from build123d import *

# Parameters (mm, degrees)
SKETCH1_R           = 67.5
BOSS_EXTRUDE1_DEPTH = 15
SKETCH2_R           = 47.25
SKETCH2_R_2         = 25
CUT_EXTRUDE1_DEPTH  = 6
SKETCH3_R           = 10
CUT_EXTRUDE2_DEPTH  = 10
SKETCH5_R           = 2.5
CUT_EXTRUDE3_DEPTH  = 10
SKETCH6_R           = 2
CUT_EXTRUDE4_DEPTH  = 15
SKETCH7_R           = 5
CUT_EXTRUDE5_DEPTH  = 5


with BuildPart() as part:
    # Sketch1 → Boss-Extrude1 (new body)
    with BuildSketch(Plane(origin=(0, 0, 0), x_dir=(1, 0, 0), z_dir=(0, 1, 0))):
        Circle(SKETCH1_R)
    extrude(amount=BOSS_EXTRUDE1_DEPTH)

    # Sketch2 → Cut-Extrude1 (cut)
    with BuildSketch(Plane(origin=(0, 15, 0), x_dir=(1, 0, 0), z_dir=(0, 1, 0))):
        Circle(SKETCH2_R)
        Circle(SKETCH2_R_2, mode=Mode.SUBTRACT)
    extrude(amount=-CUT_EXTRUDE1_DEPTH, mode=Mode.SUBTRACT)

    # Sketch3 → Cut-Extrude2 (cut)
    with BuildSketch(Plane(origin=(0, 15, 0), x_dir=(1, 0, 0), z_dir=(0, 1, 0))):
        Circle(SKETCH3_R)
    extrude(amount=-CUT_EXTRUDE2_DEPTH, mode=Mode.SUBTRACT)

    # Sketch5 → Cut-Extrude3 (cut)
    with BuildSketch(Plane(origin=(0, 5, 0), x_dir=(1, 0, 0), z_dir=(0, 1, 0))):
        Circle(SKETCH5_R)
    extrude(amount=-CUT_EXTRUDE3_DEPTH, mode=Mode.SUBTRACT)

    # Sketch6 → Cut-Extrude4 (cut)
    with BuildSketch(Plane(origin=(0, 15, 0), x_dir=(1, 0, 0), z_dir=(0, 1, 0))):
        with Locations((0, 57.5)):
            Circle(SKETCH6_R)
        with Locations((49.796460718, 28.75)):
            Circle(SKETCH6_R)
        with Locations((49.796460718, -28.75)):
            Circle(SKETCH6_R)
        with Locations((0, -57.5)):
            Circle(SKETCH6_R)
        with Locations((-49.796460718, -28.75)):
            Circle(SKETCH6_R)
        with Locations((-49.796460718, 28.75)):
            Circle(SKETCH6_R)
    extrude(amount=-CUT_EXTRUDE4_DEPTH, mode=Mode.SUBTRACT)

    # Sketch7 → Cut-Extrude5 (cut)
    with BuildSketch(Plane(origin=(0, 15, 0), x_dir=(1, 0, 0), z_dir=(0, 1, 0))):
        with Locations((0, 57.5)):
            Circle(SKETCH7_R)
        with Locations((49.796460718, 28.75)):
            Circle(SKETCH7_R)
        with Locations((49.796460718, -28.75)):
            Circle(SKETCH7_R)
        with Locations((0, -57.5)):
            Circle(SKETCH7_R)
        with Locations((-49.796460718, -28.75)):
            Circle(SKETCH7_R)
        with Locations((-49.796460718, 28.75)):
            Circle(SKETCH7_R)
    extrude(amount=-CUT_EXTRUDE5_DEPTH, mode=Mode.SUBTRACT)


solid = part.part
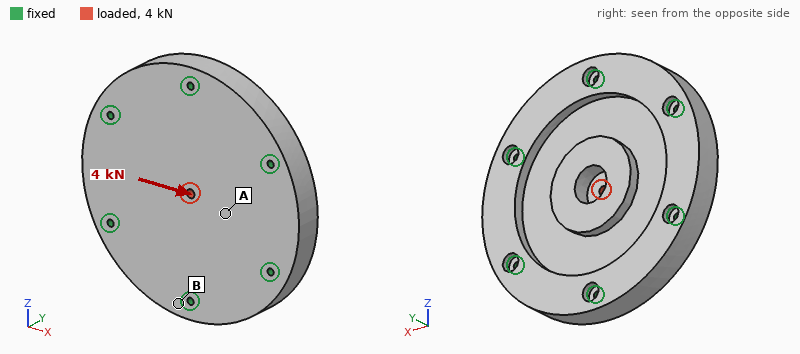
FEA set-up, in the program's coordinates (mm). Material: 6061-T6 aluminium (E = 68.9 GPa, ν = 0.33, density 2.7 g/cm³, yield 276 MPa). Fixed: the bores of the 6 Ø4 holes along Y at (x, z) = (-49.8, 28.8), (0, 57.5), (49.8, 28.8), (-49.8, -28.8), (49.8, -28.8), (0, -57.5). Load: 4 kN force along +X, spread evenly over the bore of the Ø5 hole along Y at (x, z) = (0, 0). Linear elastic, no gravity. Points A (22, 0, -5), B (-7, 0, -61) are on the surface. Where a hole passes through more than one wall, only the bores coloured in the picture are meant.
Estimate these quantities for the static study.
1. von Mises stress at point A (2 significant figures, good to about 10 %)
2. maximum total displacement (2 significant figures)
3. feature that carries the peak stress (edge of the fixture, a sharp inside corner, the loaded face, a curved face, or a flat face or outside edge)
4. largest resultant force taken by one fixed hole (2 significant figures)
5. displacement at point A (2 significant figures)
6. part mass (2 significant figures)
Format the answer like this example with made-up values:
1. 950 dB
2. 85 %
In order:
1. 7.5 MPa
2. 8.4 µm
3. the loaded face
4. 850 N
5. 2.6 µm
6. 480 g
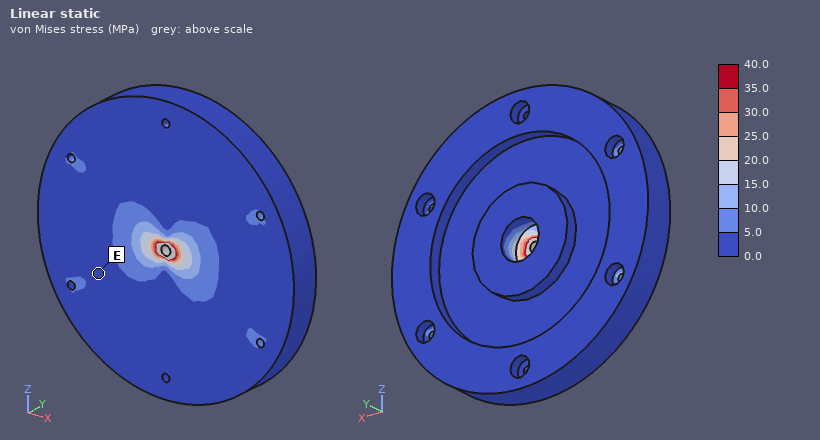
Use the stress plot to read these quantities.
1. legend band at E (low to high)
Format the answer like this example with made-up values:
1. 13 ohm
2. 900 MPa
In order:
1. 0.0 to 5.0 MPa
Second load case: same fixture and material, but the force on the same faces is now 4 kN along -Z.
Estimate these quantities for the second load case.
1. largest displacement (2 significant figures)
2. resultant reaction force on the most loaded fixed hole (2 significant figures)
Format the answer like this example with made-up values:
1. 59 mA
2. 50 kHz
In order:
1. 8.4 µm
2. 960 N
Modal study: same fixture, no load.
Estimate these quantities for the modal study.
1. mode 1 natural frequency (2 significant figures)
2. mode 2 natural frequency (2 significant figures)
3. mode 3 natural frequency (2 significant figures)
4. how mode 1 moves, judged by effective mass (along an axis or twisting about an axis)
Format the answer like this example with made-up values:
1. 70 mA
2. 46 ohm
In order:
1. 5700 Hz
2. 10 kHz
3. 10 kHz
4. along Y
